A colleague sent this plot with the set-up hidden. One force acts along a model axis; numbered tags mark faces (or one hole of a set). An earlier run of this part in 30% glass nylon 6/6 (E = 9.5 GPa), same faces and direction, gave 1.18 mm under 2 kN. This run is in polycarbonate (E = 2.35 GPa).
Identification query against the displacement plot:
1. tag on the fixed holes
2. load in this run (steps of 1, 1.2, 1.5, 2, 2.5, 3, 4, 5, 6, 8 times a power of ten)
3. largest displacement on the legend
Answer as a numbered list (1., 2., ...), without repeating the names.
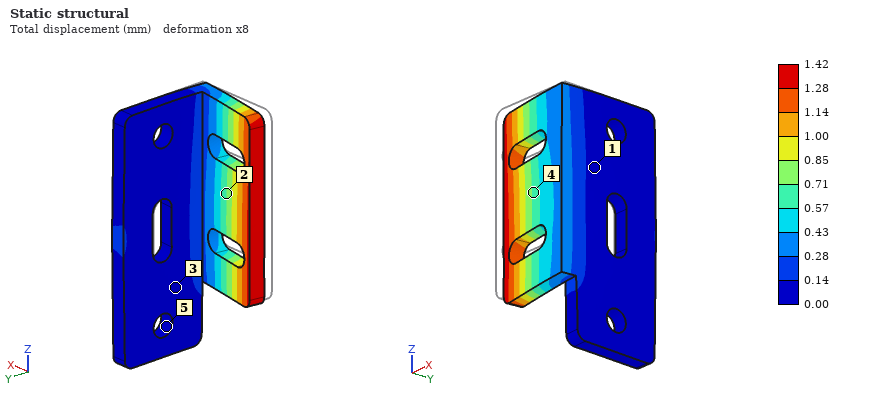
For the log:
1. 5
2. 600 N
3. 1.42 mm
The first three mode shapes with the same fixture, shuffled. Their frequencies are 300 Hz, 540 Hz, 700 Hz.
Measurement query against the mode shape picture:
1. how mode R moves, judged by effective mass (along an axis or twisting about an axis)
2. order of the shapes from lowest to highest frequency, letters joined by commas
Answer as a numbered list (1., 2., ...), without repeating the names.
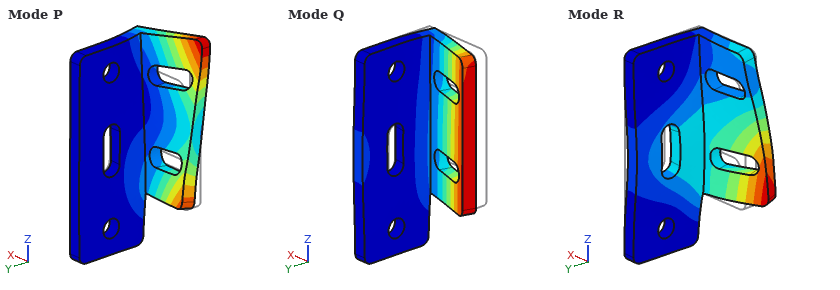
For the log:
1. along X
2. Q, P, R
